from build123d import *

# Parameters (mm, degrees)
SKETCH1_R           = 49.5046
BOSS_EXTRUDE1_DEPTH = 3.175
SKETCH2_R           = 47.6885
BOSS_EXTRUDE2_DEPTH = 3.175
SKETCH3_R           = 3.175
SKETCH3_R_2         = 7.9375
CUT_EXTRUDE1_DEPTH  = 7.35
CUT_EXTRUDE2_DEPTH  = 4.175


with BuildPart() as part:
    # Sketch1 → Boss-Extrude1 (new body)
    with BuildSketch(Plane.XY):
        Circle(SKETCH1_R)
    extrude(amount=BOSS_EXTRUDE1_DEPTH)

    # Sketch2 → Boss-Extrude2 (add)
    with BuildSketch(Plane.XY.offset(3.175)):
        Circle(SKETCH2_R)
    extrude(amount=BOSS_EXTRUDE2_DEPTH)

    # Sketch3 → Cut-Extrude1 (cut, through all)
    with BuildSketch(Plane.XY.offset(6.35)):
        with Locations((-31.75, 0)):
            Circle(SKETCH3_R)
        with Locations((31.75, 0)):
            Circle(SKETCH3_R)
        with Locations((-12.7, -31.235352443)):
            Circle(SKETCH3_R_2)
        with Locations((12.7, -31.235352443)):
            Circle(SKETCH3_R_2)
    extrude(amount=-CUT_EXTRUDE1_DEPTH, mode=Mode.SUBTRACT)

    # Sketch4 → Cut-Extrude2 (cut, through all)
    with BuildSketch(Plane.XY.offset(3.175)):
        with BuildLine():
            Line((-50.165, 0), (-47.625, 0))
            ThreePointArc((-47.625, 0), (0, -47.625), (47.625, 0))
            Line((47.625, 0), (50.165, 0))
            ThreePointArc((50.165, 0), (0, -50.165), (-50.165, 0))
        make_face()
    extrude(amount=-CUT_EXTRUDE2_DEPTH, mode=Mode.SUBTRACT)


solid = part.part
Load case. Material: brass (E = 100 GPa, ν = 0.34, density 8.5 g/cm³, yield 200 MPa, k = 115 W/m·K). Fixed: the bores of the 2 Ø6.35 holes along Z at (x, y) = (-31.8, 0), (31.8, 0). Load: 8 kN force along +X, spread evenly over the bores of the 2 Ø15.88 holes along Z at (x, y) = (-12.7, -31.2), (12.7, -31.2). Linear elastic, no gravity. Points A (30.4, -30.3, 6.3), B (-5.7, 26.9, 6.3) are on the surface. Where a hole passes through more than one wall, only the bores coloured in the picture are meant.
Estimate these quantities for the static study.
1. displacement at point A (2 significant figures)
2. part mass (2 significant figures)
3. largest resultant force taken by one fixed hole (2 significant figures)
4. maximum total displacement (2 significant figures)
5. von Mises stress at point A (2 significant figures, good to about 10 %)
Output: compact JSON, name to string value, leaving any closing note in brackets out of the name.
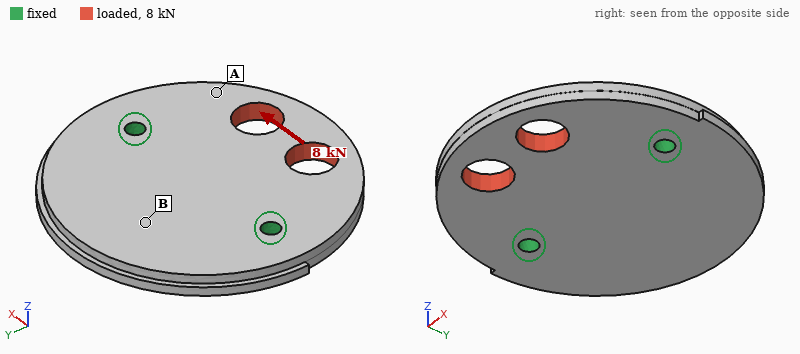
{"displacement at point A": "19 µm", "part mass": "370 g", "largest resultant force taken by one fixed hole": "5.5 kN", "maximum total displacement": "31 µm", "von Mises stress at point A": "23 MPa"}
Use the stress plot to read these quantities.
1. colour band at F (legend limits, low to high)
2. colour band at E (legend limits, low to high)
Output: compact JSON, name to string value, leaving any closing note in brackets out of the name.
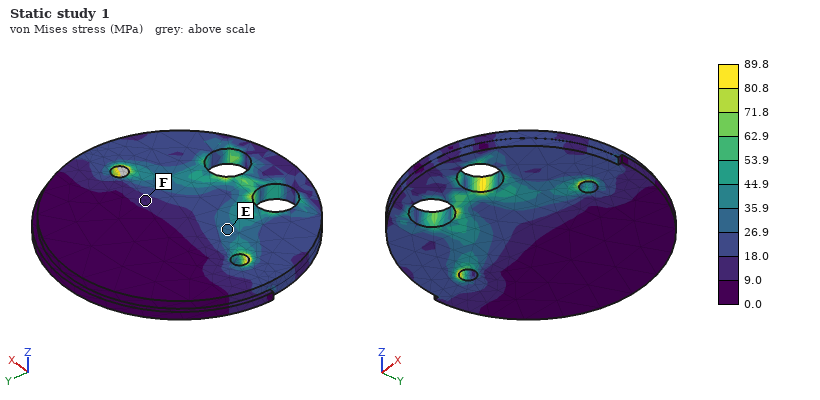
{"colour band at F": "9.0 to 18.0 MPa", "colour band at E": "26.9 to 35.9 MPa"}
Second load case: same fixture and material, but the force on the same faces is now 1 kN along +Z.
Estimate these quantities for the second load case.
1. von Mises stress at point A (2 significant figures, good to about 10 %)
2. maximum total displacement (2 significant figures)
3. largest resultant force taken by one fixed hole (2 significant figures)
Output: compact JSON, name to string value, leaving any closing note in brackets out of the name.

{"von Mises stress at point A": "20 MPa", "maximum total displacement": "0.16 mm", "largest resultant force taken by one fixed hole": "500 N"}
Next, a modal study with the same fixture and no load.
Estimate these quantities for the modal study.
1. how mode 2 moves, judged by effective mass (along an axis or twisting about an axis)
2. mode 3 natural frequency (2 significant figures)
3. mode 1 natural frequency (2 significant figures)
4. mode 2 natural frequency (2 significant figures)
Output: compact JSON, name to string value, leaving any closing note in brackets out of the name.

{"how mode 2 moves, judged by effective mass": "along Z", "mode 3 natural frequency": "3700 Hz", "mode 1 natural frequency": "1500 Hz", "mode 2 natural frequency": "2000 Hz"}
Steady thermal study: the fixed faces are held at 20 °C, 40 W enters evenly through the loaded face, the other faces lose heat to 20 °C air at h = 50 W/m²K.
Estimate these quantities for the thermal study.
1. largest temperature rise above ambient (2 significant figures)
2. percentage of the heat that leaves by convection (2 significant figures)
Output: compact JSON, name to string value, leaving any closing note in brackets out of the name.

{"largest temperature rise above ambient": "34 K", "percentage of the heat that leaves by convection": "18 %"}
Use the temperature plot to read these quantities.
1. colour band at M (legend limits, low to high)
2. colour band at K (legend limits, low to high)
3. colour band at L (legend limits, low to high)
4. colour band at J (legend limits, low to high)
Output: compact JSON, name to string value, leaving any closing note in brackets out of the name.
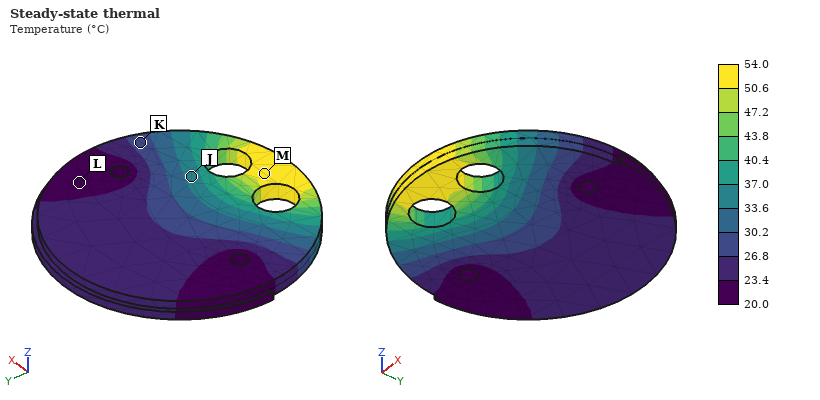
{"colour band at M": "50.6 to 54.0 °C", "colour band at K": "26.8 to 30.2 °C", "colour band at L": "20.0 to 23.4 °C", "colour band at J": "33.6 to 37.0 °C"}
